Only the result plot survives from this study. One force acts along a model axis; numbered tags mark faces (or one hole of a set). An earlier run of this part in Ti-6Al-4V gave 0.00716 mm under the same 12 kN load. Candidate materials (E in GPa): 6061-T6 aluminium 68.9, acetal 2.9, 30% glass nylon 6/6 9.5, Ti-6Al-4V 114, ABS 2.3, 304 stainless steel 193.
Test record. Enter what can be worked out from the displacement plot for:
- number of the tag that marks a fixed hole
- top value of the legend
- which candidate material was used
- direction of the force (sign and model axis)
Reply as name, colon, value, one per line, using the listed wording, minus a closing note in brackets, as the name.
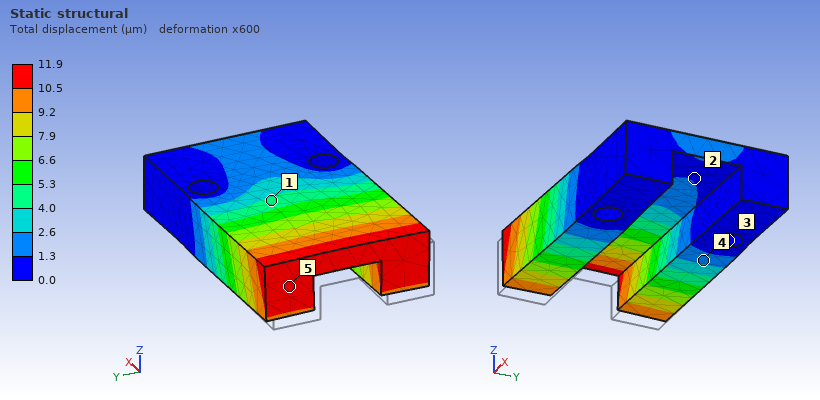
number of the tag that marks a fixed hole: 3
top value of the legend: 11.9 µm
which candidate material was used: 6061-T6 aluminium
direction of the force: +X
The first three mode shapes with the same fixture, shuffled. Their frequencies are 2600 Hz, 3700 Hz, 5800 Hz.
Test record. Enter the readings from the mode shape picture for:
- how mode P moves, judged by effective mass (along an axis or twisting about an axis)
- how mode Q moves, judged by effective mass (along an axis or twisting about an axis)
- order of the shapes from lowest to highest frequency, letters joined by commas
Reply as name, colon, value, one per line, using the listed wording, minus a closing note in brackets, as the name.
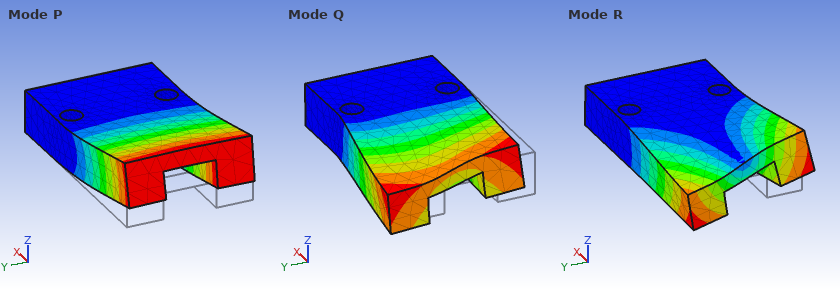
how mode P moves, judged by effective mass: along Z
how mode Q moves, judged by effective mass: along Y
order of the shapes from lowest to highest frequency, letters joined by commas: P, R, Q
